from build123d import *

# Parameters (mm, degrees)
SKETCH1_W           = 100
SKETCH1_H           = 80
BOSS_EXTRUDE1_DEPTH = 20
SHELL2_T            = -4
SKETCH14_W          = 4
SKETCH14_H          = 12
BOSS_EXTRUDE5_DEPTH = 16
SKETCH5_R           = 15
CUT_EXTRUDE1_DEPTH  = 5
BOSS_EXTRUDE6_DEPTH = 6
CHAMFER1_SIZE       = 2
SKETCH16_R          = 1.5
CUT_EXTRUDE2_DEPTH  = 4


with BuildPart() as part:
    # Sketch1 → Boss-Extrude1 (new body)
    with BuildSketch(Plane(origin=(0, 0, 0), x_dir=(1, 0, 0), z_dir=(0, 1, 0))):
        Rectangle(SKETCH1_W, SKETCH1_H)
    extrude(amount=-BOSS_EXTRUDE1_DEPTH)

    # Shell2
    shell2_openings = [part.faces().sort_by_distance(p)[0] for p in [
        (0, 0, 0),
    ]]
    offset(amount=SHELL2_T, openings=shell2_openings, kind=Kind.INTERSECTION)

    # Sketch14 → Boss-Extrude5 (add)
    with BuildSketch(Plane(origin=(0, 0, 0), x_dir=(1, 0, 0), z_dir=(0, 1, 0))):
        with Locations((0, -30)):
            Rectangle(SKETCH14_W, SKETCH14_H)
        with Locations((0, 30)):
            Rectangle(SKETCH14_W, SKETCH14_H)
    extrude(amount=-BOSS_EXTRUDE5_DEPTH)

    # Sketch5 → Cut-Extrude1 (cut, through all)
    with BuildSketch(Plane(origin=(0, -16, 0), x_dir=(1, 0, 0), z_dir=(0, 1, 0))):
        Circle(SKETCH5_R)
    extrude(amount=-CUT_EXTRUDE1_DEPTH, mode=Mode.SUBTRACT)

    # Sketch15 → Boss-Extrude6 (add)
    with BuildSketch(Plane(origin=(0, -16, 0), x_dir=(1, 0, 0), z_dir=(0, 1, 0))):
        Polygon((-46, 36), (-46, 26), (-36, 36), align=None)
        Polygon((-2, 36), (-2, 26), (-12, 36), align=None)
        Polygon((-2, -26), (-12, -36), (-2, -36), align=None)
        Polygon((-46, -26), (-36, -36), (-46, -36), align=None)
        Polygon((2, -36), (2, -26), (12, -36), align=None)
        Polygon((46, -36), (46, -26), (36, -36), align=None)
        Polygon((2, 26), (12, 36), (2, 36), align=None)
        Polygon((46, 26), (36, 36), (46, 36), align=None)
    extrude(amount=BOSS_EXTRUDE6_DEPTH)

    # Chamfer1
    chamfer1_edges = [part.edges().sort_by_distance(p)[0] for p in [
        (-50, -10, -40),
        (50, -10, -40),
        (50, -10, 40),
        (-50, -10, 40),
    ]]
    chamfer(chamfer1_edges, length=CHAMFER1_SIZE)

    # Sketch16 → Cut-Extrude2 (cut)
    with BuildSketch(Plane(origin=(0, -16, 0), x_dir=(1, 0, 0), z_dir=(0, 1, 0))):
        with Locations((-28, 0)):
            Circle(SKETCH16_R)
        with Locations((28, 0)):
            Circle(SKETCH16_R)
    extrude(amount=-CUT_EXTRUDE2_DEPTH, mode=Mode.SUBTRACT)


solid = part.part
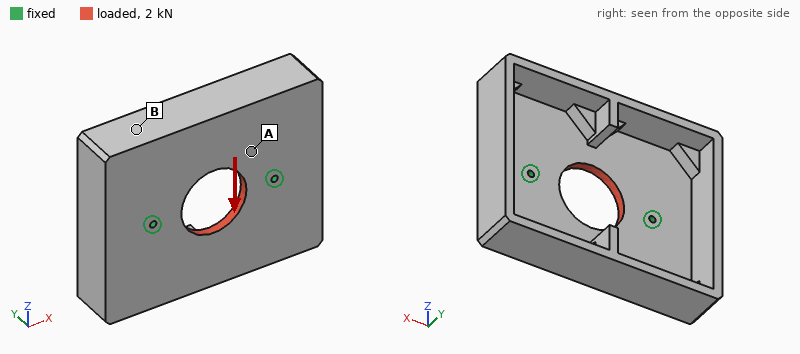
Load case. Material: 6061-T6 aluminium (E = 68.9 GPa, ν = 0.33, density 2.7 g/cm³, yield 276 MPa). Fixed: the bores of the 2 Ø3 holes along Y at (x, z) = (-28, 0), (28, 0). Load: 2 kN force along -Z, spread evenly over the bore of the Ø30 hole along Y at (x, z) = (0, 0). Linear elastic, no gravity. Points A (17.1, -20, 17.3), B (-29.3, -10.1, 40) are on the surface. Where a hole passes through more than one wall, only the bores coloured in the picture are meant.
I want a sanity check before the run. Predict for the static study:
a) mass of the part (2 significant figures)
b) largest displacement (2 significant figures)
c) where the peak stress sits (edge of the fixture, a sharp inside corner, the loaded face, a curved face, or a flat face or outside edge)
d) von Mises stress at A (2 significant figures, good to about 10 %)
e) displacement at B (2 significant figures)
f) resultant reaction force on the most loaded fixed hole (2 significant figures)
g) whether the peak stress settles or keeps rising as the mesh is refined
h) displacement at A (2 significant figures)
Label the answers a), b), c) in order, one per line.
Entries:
a) 150 g
b) 5.4 µm
c) edge of the fixture
d) 5.6 MPa
e) 2.3 µm
f) 1.0 kN
g) keeps rising
h) 3.4 µm
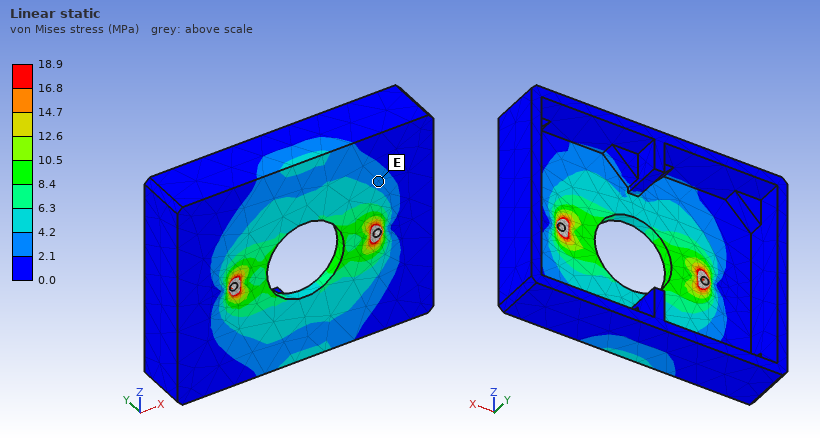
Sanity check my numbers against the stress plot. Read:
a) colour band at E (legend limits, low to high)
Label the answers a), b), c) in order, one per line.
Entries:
a) 2.1 to 4.2 MPa
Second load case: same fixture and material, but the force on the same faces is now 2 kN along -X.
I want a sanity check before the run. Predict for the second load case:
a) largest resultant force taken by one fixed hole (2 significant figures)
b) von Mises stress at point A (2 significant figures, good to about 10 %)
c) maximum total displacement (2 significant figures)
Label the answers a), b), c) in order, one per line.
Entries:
a) 1.0 kN
b) 3.6 MPa
c) 4.8 µm
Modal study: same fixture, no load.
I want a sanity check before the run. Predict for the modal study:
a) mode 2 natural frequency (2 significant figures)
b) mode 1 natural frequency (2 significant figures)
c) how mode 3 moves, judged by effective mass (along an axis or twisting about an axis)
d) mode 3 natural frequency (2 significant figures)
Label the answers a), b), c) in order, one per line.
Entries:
a) 1600 Hz
b) 810 Hz
c) along Y
d) 2100 Hz
